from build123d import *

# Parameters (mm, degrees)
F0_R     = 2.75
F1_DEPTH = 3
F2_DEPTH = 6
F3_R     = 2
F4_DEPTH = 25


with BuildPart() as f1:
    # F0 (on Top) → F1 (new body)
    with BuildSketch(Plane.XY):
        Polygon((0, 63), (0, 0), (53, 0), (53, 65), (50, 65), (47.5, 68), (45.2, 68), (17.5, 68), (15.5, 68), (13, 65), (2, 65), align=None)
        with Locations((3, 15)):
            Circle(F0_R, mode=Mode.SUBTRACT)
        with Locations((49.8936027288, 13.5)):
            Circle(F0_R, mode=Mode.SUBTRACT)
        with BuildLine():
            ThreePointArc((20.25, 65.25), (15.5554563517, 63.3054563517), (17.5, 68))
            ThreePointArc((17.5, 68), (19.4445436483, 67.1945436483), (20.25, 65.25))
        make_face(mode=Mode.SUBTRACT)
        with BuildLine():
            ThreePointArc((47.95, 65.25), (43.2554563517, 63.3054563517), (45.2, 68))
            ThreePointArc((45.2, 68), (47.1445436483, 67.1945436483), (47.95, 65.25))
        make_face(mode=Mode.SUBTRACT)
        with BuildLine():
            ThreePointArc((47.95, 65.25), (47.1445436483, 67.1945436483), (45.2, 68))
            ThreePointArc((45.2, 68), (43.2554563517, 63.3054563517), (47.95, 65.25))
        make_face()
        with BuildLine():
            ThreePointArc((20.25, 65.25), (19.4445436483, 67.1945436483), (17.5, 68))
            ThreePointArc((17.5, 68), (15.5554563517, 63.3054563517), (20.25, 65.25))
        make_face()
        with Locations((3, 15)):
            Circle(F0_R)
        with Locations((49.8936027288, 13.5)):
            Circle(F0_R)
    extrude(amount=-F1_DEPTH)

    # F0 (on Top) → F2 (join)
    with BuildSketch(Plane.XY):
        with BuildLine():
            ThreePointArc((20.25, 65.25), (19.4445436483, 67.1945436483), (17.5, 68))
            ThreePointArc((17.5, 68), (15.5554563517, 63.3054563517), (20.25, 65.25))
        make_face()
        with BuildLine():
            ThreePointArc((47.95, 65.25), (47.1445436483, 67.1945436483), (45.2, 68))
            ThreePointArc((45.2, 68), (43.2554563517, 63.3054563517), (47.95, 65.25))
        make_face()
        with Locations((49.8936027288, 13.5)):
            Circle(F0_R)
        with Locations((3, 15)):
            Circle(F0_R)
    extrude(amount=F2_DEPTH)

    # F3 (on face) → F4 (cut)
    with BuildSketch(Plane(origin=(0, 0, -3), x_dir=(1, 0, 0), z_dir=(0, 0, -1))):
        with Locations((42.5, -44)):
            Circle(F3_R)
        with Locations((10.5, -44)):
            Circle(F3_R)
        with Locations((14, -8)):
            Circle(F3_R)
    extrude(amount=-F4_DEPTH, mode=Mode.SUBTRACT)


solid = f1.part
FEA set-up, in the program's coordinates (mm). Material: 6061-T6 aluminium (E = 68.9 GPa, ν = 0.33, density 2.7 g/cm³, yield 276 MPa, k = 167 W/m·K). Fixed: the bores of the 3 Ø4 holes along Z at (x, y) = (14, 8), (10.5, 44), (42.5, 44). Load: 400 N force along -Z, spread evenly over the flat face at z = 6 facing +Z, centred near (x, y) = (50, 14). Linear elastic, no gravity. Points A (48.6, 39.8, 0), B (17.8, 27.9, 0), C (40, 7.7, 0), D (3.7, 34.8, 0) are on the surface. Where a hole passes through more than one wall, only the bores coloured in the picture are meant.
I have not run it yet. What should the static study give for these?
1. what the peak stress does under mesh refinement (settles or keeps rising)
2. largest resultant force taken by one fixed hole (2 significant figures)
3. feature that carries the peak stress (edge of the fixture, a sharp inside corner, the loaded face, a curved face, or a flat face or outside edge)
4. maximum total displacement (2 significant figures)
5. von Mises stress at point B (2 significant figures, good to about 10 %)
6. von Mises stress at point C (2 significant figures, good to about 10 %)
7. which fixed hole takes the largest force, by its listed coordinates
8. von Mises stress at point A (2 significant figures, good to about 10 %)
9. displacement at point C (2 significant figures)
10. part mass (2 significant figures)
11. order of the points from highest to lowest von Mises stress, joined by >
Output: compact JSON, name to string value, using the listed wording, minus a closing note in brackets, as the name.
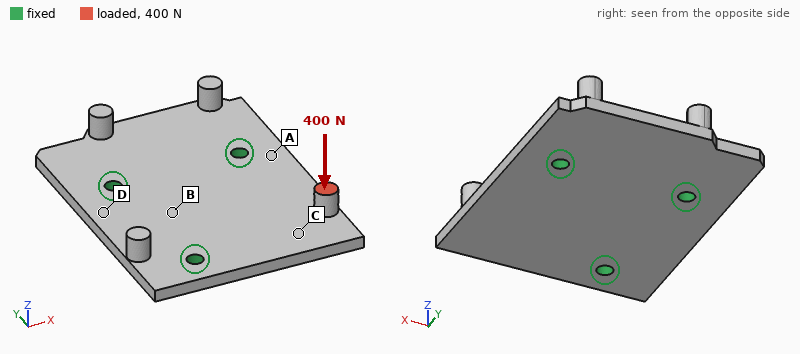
{"what the peak stress does under mesh refinement": "keeps rising", "largest resultant force taken by one fixed hole": "310 N", "feature that carries the peak stress": "edge of the fixture", "maximum total displacement": "0.63 mm", "von Mises stress at point B": "32 MPa", "von Mises stress at point C": "59 MPa", "which fixed hole takes the largest force, by its listed coordinates": "(42.5, 44)", "von Mises stress at point A": "120 MPa", "displacement at point C": "0.30 mm", "part mass": "30 g", "order of the points from highest to lowest von Mises stress, joined by >": "A > C > B > D"}
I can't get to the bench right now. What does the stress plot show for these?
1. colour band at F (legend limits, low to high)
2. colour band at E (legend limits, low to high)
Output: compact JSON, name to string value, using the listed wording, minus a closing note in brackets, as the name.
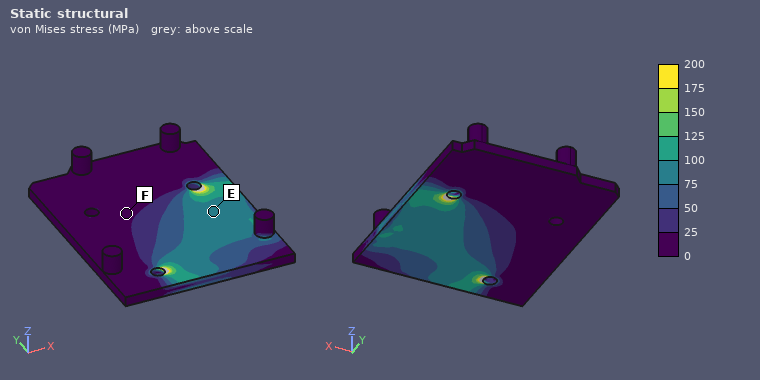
{"colour band at F": "0 to 25 MPa", "colour band at E": "75 to 100 MPa"}
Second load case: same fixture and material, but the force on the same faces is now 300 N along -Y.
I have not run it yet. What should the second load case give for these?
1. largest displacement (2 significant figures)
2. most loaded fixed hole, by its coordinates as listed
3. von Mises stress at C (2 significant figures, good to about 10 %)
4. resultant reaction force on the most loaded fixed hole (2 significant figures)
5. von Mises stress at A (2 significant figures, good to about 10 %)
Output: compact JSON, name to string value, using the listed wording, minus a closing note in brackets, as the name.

{"largest displacement": "0.18 mm", "most loaded fixed hole, by its coordinates as listed": "(42.5, 44)", "von Mises stress at C": "33 MPa", "resultant reaction force on the most loaded fixed hole": "250 N", "von Mises stress at A": "9.5 MPa"}
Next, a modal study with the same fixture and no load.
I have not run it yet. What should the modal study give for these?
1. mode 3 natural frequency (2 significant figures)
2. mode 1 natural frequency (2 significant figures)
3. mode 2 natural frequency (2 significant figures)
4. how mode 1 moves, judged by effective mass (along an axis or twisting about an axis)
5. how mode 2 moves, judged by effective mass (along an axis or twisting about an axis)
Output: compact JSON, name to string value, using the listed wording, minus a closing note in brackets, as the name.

{"mode 3 natural frequency": "6100 Hz", "mode 1 natural frequency": "2700 Hz", "mode 2 natural frequency": "3800 Hz", "how mode 1 moves, judged by effective mass": "along Z", "how mode 2 moves, judged by effective mass": "along Z"}
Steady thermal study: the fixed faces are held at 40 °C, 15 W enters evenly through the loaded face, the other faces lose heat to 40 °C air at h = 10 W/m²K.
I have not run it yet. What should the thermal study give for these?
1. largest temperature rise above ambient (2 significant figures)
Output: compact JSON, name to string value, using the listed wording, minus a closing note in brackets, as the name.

{"largest temperature rise above ambient": "54 K"}
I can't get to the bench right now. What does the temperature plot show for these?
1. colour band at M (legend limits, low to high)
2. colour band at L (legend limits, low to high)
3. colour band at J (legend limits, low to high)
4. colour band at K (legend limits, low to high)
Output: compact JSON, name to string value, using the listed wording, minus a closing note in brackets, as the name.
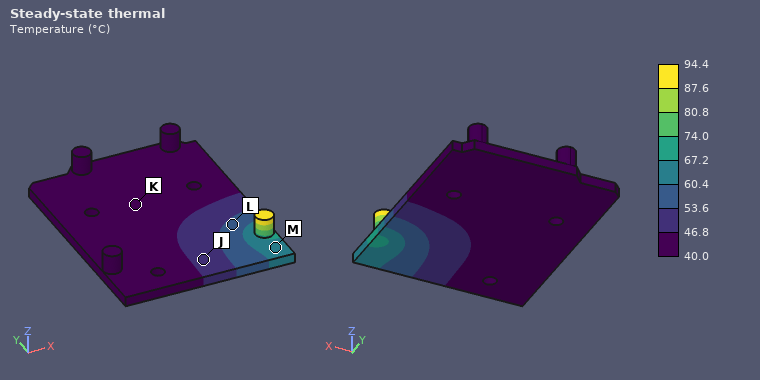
{"colour band at M": "60.4 to 67.2 °C", "colour band at L": "53.6 to 60.4 °C", "colour band at J": "46.8 to 53.6 °C", "colour band at K": "40.0 to 46.8 °C"}
